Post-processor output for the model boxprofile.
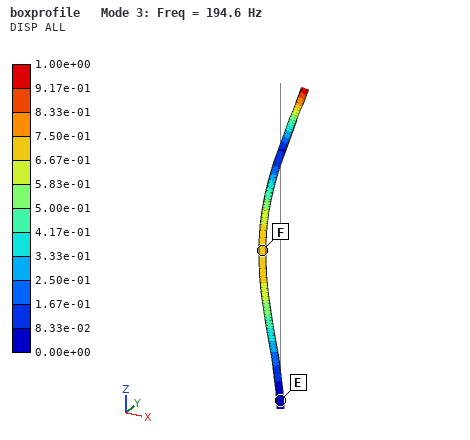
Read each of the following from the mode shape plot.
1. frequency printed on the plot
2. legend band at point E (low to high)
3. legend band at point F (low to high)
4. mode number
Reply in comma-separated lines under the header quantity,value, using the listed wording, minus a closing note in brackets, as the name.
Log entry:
quantity,value
frequency printed on the plot,194.6 Hz
legend band at point E,0.00e+00 to 8.33e-02
legend band at point F,6.67e-01 to 7.50e-01
mode number,3
